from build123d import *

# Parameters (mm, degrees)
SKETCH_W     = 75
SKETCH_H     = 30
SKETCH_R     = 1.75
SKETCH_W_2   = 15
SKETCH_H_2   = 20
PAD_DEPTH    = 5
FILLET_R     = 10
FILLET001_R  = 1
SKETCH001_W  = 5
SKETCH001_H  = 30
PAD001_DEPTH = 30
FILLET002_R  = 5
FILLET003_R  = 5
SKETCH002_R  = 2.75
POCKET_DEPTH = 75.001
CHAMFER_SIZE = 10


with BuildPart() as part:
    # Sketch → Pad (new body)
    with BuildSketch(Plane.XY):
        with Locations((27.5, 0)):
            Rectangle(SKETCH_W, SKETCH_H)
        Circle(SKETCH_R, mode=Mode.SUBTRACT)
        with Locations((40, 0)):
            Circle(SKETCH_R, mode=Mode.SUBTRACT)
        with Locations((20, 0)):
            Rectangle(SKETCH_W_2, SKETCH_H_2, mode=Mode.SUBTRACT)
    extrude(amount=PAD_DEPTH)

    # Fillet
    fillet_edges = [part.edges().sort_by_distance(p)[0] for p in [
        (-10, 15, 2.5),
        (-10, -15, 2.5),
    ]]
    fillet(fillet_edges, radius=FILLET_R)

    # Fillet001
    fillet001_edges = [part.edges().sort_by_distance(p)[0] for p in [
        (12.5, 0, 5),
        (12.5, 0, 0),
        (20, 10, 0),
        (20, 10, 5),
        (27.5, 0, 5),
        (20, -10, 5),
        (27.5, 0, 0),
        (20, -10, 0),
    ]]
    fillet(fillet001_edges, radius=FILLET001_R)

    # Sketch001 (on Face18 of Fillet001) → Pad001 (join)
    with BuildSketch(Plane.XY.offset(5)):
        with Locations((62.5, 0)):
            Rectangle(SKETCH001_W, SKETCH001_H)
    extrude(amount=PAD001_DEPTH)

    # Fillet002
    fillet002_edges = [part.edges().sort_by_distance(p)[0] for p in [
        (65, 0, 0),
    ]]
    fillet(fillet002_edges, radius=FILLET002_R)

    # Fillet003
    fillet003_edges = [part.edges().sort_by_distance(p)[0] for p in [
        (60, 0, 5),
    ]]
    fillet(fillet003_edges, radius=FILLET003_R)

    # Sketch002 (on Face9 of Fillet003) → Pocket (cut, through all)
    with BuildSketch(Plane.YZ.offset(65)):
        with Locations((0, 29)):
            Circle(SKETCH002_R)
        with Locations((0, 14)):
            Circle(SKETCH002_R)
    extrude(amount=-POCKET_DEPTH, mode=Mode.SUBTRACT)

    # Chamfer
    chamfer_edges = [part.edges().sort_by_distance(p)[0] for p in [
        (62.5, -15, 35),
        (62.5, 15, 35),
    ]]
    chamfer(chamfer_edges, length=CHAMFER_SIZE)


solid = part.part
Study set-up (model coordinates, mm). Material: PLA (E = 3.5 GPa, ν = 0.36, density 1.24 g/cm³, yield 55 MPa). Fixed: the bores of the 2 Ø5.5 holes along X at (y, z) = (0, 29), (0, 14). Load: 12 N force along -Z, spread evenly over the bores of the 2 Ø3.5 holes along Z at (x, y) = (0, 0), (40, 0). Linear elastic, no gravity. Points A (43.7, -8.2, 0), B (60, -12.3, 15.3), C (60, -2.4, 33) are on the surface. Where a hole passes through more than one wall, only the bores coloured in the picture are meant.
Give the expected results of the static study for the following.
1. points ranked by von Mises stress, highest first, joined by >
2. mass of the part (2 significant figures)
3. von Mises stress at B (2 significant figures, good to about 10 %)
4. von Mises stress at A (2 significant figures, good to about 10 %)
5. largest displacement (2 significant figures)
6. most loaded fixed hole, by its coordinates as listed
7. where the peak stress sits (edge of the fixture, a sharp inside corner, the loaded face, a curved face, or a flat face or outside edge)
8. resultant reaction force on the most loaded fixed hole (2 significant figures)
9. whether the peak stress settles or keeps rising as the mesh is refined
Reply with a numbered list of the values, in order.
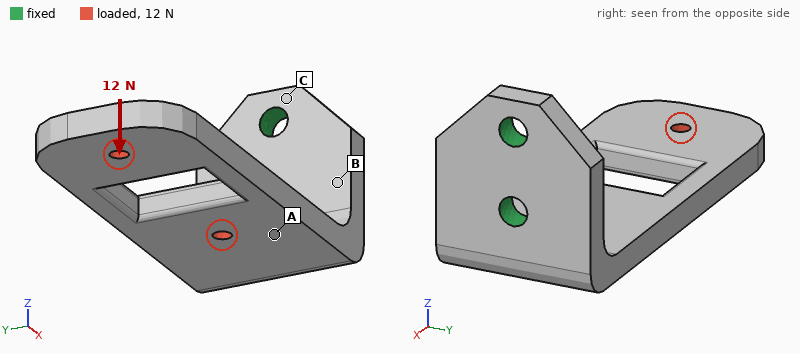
1. A > B > C
2. 16 g
3. 1.6 MPa
4. 2.3 MPa
5. 0.98 mm
6. (0, 14)
7. edge of the fixture
8. 17 N
9. keeps rising
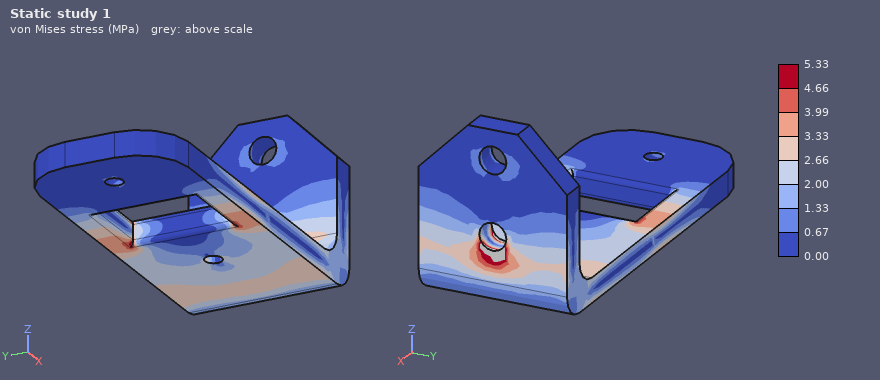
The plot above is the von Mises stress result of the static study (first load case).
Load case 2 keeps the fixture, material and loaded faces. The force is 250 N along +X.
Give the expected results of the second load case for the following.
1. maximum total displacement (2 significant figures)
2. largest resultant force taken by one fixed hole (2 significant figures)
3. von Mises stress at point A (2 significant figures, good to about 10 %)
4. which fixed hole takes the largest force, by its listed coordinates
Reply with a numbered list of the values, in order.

1. 1.0 mm
2. 300 N
3. 1.5 MPa
4. (0, 14)
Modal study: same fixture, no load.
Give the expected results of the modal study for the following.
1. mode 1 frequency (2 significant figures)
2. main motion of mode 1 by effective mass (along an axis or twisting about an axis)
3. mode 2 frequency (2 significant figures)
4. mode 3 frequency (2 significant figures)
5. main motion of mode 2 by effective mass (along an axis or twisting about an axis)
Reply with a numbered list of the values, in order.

1. 240 Hz
2. along Z
3. 480 Hz
4. 1100 Hz
5. along Y
